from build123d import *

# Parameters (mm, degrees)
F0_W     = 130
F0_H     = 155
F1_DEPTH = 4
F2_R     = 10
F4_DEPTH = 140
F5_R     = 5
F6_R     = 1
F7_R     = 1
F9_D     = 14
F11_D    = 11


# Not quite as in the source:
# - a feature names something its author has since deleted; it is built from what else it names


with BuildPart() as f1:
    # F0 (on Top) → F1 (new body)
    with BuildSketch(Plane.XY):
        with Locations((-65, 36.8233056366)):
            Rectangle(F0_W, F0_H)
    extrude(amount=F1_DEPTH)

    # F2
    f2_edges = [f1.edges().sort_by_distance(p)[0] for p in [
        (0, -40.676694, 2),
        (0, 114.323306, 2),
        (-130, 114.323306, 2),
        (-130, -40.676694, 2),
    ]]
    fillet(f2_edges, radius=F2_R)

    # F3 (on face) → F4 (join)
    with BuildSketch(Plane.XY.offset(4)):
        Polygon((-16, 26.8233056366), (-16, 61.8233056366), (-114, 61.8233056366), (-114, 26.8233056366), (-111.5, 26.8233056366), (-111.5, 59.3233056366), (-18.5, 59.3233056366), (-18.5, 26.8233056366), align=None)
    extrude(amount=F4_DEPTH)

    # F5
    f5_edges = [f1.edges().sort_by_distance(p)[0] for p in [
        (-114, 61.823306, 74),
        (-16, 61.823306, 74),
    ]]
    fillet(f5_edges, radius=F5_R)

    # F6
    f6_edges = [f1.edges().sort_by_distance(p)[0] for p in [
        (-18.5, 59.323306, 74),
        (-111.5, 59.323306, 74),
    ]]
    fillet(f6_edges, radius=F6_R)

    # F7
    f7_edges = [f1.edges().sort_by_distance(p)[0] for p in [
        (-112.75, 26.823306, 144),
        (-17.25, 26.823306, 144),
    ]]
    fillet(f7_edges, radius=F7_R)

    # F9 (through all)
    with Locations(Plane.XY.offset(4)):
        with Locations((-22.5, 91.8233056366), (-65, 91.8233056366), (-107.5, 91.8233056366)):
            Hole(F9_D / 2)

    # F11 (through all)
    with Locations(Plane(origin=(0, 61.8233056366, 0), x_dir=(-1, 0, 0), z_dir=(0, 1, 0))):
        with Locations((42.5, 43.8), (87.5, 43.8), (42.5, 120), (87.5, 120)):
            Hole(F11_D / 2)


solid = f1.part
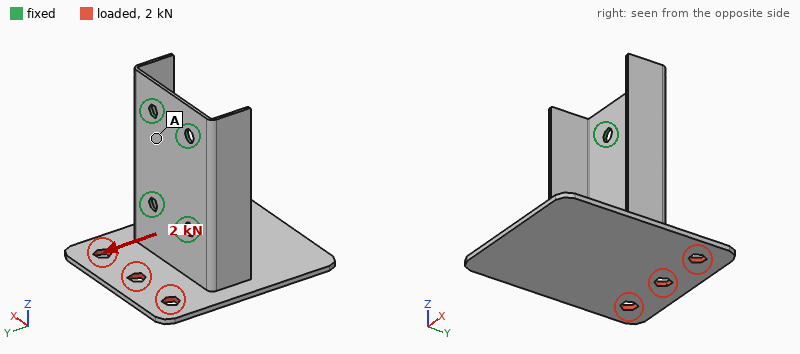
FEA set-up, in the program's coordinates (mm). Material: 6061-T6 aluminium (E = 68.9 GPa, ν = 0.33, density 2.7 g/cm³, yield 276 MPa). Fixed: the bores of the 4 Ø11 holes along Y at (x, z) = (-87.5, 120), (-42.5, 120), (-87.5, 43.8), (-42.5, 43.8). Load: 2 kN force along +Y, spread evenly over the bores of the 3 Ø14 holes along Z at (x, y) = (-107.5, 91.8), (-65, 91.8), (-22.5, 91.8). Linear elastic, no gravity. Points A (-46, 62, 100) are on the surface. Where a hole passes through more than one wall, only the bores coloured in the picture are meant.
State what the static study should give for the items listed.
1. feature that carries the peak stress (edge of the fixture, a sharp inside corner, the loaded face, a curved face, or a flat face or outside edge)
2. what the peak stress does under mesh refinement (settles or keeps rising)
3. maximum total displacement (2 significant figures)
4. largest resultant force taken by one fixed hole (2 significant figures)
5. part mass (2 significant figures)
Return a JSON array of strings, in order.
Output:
["edge of the fixture", "keeps rising", "1.2 mm", "1.5 kN", "360 g"]
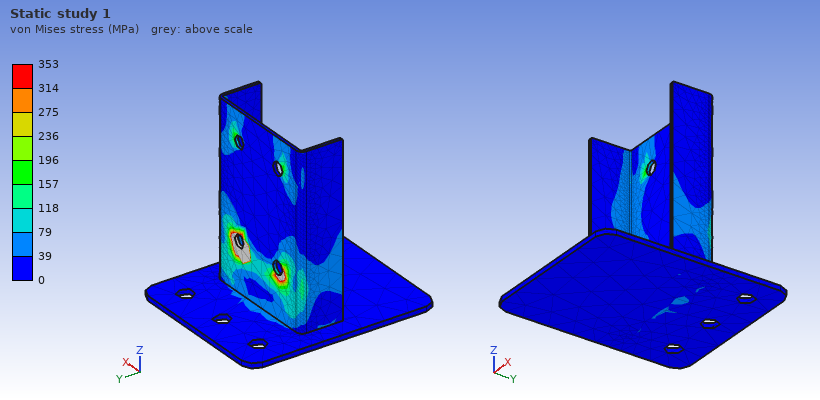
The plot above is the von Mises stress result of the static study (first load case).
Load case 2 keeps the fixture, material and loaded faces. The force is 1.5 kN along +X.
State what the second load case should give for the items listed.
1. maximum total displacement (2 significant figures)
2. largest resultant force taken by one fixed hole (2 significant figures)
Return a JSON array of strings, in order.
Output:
["1.4 mm", "1.3 kN"]
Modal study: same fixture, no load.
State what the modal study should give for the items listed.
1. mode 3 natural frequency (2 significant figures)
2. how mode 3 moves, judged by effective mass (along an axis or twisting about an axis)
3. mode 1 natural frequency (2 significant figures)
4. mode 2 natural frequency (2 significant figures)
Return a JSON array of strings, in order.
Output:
["620 Hz", "along Y", "330 Hz", "380 Hz"]
